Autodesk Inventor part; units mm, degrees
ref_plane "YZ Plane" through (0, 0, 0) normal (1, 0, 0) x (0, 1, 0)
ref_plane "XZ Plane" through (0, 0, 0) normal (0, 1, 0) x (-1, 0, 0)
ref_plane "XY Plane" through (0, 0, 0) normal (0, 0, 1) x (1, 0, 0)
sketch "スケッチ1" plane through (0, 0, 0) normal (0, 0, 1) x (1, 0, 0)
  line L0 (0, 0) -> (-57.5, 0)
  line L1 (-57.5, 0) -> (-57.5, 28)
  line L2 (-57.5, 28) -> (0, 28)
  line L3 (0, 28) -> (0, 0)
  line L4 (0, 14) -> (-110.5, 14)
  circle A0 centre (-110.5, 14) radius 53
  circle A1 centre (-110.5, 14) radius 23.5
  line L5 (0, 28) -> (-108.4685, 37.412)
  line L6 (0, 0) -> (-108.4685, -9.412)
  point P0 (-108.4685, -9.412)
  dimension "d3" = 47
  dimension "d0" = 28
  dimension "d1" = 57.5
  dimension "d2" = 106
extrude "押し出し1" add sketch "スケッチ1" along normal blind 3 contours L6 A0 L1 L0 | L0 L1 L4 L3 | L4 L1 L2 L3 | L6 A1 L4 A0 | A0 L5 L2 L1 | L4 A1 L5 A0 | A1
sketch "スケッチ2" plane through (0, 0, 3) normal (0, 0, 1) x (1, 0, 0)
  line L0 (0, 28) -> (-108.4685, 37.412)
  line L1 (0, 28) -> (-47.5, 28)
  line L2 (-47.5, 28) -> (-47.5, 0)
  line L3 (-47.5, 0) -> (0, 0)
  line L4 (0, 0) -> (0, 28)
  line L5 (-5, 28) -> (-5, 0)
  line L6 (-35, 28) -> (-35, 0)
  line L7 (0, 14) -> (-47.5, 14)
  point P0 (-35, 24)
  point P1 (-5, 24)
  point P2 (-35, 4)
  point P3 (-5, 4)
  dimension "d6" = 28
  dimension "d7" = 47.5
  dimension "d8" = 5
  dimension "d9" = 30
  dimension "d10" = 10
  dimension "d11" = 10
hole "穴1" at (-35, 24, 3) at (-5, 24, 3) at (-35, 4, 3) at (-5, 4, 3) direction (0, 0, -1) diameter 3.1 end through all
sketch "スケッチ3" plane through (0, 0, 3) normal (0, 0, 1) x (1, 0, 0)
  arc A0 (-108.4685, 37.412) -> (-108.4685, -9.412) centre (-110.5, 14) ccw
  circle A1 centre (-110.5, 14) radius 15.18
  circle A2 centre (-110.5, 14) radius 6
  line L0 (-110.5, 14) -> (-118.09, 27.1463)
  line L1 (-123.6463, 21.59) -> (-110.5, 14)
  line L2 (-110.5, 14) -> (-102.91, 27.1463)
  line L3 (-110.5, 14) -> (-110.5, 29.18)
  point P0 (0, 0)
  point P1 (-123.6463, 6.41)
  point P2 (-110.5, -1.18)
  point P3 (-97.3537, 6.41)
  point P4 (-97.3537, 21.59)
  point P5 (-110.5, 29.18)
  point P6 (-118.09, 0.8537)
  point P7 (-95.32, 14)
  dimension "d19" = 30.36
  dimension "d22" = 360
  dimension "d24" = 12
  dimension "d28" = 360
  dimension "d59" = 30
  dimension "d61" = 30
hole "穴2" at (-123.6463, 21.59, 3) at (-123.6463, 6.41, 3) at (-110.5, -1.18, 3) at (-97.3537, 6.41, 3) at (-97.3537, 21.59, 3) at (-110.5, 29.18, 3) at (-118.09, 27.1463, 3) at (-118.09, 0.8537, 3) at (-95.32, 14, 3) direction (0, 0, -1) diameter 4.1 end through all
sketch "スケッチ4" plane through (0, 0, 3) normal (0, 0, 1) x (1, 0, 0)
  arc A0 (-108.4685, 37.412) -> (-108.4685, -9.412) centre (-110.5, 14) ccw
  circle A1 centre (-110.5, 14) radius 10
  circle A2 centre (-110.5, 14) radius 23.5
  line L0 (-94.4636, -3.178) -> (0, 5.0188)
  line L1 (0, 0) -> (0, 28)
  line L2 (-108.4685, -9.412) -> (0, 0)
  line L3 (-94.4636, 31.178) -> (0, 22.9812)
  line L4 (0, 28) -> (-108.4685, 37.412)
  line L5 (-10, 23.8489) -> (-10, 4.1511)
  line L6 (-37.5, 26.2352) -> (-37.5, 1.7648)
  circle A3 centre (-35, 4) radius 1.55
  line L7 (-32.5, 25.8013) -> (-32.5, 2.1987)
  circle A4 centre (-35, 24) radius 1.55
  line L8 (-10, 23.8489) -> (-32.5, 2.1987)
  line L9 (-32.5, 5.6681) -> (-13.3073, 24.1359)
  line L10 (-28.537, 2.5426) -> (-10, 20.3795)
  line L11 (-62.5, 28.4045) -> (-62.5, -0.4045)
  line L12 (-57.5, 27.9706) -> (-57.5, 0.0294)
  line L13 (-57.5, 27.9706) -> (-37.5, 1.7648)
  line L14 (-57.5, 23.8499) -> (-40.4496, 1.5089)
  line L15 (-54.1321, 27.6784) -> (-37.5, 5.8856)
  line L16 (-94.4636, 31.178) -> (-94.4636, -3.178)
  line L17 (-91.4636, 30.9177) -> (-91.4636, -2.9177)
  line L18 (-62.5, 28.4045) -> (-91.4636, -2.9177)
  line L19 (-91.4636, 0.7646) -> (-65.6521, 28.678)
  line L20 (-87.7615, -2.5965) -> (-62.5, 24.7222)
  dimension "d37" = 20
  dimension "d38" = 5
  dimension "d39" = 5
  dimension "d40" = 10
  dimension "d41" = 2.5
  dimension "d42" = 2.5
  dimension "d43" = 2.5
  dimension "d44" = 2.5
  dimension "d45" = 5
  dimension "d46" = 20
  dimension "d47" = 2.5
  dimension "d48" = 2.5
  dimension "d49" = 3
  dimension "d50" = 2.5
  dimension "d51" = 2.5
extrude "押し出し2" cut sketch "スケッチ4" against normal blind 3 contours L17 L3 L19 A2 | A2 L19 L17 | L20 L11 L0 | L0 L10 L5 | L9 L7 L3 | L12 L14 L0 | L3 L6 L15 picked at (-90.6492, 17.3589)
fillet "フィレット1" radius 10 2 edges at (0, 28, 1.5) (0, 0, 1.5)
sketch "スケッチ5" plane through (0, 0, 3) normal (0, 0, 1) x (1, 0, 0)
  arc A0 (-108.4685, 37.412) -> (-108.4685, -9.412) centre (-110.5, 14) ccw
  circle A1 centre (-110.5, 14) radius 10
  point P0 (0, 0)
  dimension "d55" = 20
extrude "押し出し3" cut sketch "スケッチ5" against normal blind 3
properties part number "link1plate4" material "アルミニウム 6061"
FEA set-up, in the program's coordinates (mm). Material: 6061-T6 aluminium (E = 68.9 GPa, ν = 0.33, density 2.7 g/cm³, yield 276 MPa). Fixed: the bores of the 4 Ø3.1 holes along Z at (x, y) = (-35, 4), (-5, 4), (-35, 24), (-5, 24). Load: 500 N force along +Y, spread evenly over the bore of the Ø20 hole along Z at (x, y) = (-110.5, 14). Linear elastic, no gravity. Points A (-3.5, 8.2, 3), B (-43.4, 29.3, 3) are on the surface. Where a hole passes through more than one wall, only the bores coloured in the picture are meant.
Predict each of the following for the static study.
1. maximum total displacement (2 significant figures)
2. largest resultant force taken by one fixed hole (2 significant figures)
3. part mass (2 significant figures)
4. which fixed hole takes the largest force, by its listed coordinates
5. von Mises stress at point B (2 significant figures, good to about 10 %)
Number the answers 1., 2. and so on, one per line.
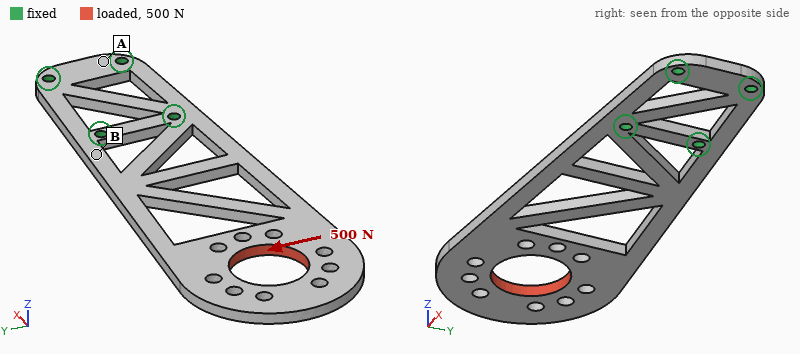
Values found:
1. 0.38 mm
2. 1.2 kN
3. 25 g
4. (-35, 4)
5. 85 MPa
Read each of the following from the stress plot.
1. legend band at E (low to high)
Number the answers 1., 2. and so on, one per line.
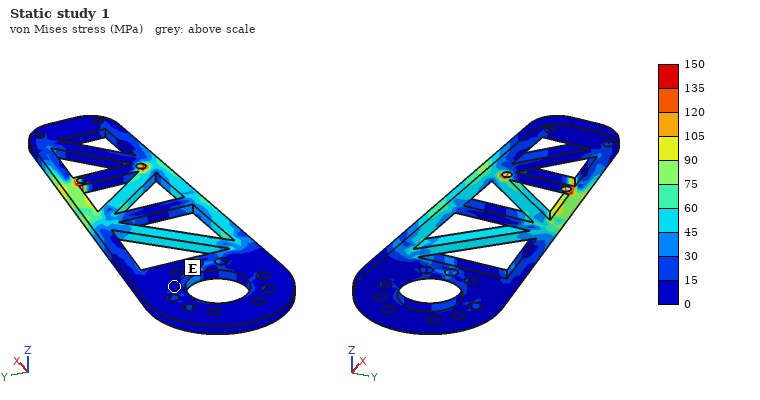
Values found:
1. 0 to 15 MPa
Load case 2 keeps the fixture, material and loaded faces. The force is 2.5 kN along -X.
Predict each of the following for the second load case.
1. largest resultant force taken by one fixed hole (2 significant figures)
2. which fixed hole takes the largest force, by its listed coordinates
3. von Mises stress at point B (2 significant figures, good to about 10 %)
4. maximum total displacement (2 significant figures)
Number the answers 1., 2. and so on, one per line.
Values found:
1. 1.1 kN
2. (-35, 4)
3. 79 MPa
4. 0.10 mm
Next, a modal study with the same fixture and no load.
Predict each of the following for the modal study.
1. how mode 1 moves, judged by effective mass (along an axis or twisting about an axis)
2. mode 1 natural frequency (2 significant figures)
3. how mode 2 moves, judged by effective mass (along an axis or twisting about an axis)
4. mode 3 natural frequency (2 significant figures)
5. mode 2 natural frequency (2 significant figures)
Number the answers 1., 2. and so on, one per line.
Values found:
1. along Z
2. 180 Hz
3. twisting about X
4. 1300 Hz
5. 800 Hz
